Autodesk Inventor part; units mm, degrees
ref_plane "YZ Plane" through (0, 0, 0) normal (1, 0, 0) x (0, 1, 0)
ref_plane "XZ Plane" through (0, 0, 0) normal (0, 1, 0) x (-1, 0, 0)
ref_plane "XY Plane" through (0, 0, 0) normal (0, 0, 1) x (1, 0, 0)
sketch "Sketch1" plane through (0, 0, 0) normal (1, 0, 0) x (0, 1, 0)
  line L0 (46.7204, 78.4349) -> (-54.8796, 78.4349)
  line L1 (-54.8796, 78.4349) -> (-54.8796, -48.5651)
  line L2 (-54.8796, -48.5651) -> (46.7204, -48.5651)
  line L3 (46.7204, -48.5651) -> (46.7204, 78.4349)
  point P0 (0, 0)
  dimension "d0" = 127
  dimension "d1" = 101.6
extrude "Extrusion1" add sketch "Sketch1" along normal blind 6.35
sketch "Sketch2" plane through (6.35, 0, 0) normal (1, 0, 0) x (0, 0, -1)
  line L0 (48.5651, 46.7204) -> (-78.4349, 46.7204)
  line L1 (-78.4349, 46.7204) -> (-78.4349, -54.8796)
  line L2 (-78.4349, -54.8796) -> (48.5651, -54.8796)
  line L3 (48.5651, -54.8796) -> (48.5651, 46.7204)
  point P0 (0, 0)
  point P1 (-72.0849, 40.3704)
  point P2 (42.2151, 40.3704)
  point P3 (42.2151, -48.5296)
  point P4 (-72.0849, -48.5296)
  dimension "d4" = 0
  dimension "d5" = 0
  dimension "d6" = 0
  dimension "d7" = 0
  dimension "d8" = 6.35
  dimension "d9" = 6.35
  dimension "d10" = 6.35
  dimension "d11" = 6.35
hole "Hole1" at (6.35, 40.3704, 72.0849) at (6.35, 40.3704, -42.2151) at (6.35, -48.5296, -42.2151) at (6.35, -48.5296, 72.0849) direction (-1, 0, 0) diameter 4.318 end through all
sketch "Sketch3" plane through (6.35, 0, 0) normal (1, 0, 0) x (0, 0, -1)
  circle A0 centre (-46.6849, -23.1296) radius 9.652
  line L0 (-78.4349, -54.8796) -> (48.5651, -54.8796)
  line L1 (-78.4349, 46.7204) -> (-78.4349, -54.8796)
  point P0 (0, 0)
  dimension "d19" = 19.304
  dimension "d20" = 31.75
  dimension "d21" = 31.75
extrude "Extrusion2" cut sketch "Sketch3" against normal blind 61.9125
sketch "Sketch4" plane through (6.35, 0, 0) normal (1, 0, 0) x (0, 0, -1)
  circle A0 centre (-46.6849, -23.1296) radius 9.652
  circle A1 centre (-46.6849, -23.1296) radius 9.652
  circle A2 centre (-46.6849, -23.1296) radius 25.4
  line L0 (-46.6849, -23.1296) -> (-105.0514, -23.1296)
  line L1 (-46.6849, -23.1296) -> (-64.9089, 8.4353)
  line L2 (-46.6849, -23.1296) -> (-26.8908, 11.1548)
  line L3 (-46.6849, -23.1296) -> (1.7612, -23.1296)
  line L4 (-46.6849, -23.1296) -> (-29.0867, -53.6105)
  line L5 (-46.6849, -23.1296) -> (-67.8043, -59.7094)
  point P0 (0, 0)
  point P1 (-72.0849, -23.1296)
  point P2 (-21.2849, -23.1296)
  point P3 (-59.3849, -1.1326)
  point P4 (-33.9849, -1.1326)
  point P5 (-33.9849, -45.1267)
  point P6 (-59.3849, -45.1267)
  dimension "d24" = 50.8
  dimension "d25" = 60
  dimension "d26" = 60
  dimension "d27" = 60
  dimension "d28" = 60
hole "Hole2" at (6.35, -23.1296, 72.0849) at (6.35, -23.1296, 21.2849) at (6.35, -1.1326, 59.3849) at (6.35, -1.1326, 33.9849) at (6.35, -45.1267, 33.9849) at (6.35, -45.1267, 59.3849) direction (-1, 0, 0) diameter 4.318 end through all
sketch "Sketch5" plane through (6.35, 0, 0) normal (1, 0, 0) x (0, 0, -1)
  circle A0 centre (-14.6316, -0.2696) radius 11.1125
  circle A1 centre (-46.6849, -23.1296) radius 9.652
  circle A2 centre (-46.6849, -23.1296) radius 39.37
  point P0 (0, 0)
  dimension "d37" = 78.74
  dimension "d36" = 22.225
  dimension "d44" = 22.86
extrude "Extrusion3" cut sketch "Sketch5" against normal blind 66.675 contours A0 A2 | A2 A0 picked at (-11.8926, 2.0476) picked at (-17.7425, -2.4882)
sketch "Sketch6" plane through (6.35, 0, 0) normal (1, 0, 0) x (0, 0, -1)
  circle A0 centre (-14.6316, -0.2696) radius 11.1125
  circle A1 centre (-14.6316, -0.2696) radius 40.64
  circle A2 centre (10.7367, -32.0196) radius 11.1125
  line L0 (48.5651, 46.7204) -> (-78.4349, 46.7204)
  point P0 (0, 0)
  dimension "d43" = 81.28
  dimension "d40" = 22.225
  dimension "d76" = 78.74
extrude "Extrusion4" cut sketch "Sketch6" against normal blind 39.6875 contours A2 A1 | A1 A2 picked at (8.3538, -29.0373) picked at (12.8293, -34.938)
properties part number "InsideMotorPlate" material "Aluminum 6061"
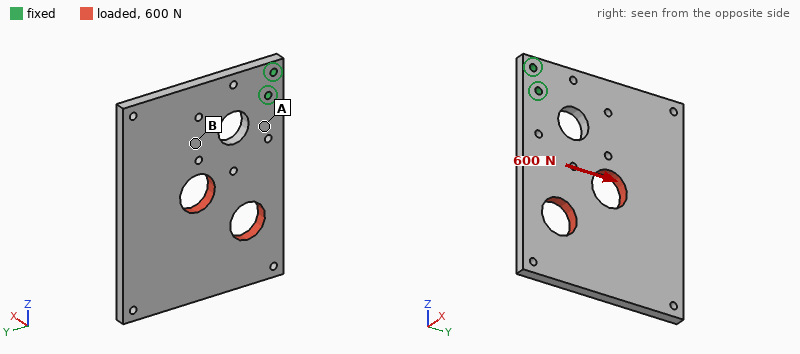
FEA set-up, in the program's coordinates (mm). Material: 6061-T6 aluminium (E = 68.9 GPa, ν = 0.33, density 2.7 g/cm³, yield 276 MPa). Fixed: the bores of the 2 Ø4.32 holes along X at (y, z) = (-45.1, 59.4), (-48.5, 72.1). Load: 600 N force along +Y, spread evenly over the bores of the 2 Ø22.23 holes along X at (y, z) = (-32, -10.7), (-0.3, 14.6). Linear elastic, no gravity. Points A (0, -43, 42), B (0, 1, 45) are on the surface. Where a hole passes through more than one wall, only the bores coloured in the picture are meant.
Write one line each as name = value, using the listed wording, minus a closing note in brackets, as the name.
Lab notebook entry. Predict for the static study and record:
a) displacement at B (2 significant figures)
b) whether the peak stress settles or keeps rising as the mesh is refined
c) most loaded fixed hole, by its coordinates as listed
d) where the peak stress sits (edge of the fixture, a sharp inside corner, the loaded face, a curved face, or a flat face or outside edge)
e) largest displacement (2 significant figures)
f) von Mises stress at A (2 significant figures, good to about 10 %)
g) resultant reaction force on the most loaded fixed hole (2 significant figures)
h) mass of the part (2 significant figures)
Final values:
displacement at B = 0.049 mm
whether the peak stress settles or keeps rising as the mesh is refined = keeps rising
most loaded fixed hole, by its coordinates as listed = (-45.1, 59.4)
where the peak stress sits = edge of the fixture
largest displacement = 0.15 mm
von Mises stress at A = 12 MPa
resultant reaction force on the most loaded fixed hole = 2.6 kN
mass of the part = 200 g
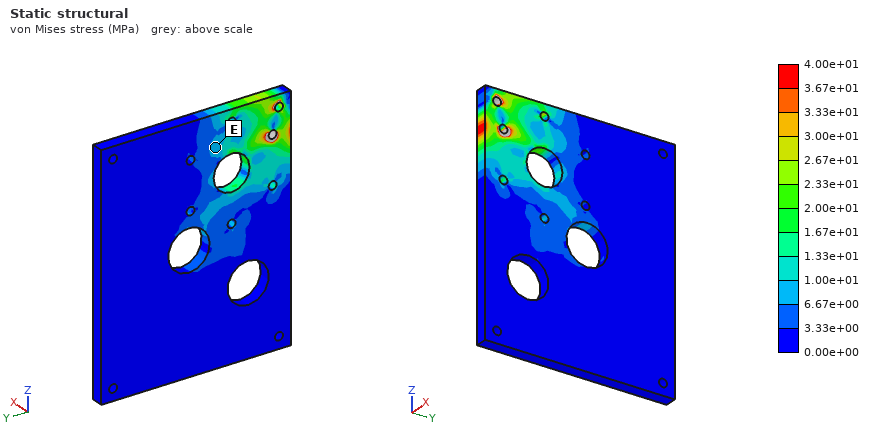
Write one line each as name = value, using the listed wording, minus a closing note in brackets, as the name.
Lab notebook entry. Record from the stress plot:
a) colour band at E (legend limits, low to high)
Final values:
colour band at E = 6.67e+00 to 1.00e+01 MPa
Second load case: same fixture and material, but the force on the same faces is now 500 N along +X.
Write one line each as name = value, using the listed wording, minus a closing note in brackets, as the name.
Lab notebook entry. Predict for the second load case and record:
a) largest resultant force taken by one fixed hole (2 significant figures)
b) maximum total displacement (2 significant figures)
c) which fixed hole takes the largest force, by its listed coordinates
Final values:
largest resultant force taken by one fixed hole = 1.5 kN
maximum total displacement = 1.9 mm
which fixed hole takes the largest force, by its listed coordinates = (-45.1, 59.4)
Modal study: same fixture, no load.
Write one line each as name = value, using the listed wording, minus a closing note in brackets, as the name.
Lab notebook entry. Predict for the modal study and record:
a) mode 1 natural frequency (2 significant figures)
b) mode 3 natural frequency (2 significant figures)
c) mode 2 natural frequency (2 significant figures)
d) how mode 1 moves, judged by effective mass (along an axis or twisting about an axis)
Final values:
mode 1 natural frequency = 240 Hz
mode 3 natural frequency = 840 Hz
mode 2 natural frequency = 490 Hz
how mode 1 moves, judged by effective mass = along X
